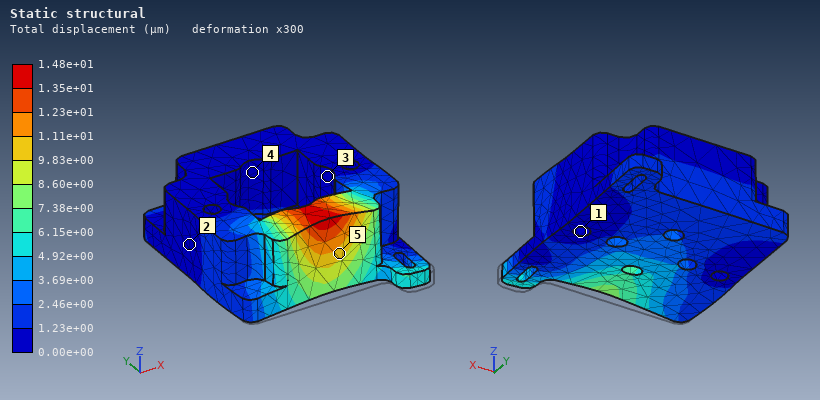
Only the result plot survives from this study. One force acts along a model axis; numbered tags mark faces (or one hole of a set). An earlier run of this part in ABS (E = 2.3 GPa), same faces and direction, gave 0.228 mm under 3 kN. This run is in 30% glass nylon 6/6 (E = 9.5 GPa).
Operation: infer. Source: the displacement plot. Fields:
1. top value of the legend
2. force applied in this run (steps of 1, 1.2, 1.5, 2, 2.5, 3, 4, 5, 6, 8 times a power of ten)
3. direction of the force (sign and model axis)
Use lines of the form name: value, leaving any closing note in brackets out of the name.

top value of the legend: 1.48e+01 µm
force applied in this run: 800 N
direction of the force: +Y
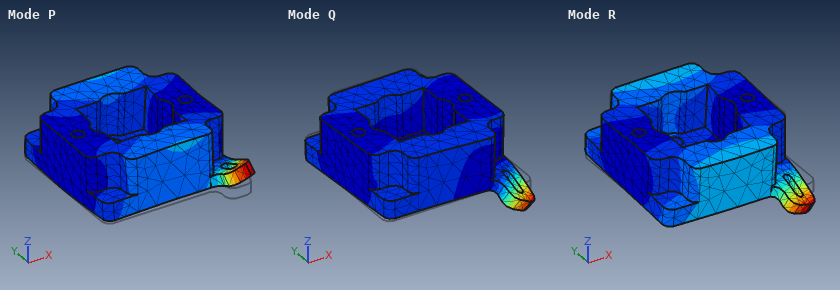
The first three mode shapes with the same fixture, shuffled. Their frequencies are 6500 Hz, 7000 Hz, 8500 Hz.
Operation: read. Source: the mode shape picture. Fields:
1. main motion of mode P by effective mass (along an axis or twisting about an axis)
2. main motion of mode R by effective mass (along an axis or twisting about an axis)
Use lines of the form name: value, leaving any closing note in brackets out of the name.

main motion of mode P by effective mass: along Z
main motion of mode R by effective mass: twisting about X
